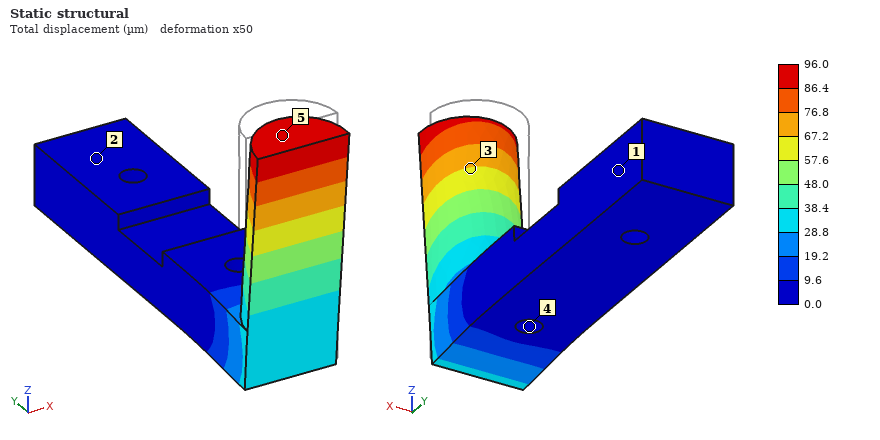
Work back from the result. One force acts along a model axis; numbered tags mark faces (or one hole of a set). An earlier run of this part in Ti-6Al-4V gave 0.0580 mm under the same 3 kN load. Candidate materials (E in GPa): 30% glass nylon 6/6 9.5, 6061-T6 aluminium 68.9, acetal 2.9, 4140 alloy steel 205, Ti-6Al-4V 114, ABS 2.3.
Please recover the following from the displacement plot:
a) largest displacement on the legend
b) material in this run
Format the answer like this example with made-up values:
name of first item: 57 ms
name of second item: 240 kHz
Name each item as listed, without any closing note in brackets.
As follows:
largest displacement on the legend: 96.0 µm
material in this run: 6061-T6 aluminium
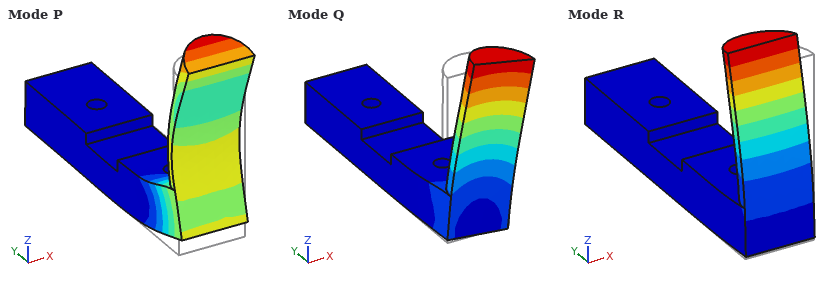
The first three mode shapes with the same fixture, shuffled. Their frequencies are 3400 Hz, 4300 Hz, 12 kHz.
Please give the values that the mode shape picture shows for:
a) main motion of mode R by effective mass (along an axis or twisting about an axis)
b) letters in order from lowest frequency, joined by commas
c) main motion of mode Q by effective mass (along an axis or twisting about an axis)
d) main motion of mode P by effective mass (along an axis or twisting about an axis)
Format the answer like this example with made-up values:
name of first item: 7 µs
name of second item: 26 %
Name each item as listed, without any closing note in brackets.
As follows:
main motion of mode R by effective mass: along Y
letters in order from lowest frequency, joined by commas: R, Q, P
main motion of mode Q by effective mass: along X
main motion of mode P by effective mass: along Z
